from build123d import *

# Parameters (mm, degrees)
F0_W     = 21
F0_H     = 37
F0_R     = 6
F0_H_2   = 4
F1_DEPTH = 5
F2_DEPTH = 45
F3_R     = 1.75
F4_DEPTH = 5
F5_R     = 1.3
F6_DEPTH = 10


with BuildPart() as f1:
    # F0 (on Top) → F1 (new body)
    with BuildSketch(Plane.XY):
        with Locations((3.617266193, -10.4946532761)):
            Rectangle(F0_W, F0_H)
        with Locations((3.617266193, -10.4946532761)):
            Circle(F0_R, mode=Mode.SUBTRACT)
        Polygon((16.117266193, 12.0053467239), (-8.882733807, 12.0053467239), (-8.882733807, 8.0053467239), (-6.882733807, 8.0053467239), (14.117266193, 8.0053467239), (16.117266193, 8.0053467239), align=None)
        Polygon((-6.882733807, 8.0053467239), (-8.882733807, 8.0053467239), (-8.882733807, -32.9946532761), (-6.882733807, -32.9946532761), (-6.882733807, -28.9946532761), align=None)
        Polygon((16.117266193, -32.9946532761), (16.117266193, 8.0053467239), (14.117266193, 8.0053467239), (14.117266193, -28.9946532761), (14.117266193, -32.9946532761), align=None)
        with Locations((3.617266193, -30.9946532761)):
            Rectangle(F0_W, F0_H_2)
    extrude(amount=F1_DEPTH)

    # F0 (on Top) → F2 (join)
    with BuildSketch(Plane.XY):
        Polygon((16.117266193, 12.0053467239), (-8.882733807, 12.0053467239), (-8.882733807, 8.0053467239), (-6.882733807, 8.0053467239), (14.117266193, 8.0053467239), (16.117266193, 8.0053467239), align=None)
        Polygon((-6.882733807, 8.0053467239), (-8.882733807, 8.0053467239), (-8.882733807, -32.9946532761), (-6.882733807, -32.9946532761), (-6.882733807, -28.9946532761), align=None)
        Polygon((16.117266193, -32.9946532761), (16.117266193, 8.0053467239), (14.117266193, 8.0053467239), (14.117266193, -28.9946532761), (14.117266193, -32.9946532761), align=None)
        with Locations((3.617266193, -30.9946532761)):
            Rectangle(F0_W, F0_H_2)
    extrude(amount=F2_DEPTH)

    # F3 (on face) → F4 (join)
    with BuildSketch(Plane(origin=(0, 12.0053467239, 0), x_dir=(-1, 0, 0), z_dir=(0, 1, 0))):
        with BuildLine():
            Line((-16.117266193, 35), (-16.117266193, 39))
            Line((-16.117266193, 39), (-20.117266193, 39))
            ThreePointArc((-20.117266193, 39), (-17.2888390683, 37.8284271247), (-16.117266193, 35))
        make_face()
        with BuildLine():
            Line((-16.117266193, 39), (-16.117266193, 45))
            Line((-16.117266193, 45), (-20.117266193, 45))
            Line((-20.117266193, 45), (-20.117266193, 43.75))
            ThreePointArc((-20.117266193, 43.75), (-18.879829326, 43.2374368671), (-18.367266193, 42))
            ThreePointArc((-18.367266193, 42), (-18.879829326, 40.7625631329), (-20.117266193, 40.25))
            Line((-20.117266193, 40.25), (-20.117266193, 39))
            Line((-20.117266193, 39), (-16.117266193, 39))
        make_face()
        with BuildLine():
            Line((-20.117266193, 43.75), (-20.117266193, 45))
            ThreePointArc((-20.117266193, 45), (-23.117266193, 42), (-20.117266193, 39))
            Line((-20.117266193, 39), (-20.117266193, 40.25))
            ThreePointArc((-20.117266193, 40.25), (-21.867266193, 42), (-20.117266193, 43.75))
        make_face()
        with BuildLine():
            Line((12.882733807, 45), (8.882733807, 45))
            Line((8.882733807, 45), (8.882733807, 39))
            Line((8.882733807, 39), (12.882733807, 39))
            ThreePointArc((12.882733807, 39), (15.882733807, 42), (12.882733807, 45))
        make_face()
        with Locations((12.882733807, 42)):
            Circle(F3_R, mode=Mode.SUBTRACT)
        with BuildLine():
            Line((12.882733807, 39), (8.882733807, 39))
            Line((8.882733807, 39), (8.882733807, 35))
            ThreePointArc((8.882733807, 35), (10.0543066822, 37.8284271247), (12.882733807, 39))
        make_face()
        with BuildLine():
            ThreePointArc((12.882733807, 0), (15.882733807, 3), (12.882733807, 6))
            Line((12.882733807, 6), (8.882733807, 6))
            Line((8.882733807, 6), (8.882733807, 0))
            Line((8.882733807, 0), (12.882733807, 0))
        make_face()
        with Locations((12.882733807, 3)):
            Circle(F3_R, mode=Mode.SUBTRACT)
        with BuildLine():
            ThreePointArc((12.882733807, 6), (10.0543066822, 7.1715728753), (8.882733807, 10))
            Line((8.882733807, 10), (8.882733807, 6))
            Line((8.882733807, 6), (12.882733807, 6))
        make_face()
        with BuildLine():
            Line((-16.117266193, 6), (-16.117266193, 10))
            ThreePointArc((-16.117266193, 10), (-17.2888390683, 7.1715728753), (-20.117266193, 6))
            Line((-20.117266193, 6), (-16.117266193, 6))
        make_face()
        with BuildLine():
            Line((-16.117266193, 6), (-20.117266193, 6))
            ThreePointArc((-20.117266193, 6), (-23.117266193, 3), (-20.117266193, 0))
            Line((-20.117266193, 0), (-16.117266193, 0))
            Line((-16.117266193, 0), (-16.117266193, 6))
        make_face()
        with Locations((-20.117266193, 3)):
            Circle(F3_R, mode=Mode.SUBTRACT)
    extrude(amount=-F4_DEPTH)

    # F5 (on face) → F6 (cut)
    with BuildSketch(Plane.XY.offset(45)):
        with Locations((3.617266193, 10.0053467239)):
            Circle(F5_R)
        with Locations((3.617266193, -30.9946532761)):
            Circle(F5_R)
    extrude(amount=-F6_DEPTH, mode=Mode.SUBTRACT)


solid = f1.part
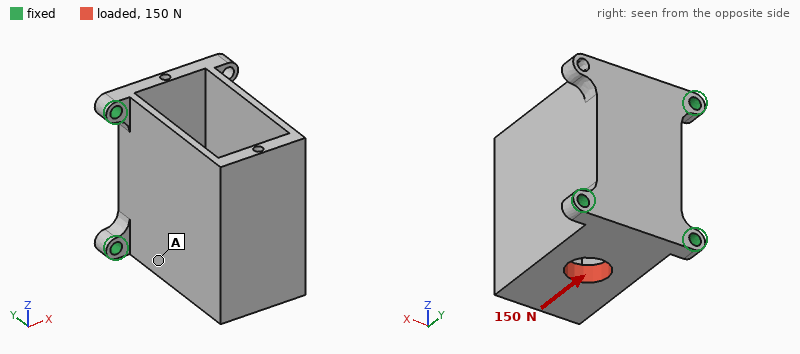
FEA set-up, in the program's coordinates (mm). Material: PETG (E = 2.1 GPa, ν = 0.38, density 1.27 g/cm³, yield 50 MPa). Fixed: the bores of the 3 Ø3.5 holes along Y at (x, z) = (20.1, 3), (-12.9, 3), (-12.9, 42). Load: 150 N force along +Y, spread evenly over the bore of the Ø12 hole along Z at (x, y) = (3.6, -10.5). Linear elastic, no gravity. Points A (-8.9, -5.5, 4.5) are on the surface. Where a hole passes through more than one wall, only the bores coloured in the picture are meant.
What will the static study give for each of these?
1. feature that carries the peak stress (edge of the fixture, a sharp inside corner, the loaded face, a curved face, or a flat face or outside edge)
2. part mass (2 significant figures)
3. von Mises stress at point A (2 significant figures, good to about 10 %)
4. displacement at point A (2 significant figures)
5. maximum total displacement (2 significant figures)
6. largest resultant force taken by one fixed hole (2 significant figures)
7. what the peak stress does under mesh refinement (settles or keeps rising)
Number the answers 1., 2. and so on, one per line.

1. edge of the fixture
2. 25 g
3. 0.86 MPa
4. 29 µm
5. 56 µm
6. 81 N
7. keeps rising
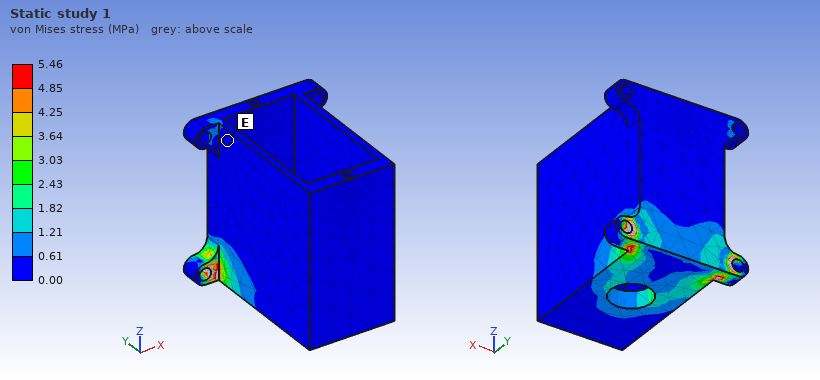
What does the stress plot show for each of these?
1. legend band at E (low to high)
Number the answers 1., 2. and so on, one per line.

1. 0.00 to 0.61 MPa
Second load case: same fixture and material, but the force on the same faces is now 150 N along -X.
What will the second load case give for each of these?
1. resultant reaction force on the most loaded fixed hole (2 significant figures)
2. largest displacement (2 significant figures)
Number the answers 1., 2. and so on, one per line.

1. 130 N
2. 0.20 mm
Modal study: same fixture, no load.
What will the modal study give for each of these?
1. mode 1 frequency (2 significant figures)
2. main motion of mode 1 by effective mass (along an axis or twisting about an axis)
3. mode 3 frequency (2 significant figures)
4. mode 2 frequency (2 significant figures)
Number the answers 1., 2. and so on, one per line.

1. 540 Hz
2. along X
3. 1800 Hz
4. 880 Hz
